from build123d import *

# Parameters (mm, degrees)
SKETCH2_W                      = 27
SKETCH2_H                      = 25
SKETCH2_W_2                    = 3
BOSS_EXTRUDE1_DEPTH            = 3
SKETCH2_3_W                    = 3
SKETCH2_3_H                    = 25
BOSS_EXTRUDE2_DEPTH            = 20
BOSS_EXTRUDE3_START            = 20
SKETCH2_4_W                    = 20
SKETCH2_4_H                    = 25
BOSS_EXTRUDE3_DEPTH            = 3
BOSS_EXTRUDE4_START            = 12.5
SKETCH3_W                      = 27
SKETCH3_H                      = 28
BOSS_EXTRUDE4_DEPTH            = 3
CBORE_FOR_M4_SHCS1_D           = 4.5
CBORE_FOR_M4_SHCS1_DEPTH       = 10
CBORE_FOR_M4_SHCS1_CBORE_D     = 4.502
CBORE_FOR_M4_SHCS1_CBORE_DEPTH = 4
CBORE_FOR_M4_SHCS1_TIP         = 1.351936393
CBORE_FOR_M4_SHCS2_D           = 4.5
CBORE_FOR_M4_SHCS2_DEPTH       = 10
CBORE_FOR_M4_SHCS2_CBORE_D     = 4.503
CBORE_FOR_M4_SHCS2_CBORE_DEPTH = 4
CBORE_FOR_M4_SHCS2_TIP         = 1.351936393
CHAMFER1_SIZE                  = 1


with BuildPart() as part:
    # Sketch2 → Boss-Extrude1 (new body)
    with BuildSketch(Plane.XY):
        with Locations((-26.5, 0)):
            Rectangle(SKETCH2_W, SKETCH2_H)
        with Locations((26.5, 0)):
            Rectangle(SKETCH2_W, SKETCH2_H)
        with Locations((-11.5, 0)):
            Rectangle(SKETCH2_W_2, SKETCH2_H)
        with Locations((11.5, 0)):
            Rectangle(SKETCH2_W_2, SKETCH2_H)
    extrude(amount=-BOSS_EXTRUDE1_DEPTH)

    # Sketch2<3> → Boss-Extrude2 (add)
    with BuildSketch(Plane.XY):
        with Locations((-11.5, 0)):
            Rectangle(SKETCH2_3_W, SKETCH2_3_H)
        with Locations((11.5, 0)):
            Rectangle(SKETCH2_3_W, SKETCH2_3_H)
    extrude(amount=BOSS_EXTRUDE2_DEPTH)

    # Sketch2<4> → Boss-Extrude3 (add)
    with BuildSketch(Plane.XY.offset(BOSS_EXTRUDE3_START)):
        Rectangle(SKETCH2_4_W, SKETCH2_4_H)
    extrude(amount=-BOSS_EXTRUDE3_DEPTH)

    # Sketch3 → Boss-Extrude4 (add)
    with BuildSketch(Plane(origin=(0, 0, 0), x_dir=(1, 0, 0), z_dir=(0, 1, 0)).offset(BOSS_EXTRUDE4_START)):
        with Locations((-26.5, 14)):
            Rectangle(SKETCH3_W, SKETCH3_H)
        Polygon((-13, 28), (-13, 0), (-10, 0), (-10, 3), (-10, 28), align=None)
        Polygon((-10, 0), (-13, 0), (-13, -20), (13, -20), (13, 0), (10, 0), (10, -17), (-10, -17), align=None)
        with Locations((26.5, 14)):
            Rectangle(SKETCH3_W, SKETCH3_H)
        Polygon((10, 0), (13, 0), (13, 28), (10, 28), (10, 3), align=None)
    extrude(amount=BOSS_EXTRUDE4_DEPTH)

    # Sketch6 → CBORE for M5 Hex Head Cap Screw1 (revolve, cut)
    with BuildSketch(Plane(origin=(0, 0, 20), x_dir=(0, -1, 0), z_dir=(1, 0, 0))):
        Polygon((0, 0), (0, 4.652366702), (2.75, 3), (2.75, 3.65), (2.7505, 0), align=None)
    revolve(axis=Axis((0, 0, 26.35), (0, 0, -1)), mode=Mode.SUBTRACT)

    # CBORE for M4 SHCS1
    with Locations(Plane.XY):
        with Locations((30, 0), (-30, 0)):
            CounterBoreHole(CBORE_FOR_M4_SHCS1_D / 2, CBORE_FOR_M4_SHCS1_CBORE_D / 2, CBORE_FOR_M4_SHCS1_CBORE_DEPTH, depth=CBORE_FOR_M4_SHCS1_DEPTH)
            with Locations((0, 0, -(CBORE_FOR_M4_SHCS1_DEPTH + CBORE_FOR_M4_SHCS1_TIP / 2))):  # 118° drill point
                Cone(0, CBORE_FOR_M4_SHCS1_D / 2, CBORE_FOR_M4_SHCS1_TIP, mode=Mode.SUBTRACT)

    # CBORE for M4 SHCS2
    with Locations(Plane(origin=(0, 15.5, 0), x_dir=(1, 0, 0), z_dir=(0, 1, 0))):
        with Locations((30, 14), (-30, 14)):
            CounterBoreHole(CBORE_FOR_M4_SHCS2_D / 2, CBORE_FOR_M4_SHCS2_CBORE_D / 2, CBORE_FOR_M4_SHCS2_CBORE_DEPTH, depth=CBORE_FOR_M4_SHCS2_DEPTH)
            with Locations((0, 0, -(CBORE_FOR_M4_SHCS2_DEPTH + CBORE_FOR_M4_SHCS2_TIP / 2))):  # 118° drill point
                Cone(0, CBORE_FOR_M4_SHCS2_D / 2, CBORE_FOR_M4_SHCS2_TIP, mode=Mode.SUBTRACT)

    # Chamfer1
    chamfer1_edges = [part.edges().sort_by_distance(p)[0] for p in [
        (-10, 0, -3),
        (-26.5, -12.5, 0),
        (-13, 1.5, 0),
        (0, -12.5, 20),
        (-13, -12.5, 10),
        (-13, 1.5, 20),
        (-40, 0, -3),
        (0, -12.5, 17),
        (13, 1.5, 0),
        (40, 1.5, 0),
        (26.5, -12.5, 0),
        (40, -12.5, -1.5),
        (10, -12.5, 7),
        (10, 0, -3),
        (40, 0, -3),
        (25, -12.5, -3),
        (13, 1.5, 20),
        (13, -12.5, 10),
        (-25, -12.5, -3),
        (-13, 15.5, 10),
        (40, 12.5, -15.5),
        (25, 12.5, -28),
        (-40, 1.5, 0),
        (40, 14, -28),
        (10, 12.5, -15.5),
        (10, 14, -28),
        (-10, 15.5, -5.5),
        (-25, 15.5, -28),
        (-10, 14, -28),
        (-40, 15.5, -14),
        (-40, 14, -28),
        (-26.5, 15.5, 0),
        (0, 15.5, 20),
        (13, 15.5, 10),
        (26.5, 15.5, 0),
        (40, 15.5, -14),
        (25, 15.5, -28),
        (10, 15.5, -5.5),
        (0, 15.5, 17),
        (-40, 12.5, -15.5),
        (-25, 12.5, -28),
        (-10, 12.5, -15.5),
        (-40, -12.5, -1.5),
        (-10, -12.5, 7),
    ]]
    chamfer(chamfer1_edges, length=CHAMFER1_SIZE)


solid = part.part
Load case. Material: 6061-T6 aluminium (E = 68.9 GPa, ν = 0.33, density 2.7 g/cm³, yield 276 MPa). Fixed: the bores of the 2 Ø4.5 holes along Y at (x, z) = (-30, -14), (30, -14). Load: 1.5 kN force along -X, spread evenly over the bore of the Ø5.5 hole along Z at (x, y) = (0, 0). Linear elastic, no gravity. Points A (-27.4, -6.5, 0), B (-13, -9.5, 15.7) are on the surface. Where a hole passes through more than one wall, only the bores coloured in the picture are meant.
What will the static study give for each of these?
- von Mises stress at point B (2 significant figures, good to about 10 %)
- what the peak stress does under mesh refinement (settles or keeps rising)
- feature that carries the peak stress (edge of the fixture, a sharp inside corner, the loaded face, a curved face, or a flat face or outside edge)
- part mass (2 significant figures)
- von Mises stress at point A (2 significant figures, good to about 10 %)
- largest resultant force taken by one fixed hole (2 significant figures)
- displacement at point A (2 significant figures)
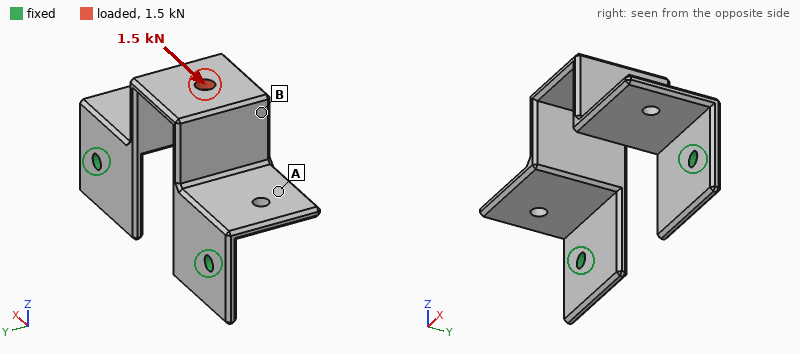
110 MPa
keeps rising
a sharp inside corner
37 g
29 MPa
1.1 kN
0.074 mm
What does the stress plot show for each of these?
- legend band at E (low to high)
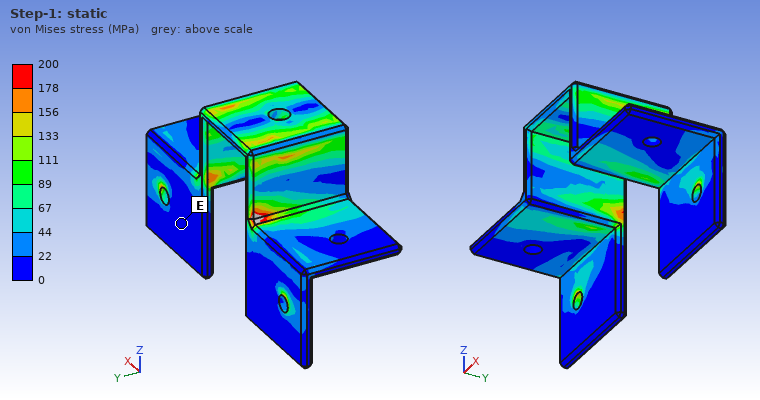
0 to 22 MPa
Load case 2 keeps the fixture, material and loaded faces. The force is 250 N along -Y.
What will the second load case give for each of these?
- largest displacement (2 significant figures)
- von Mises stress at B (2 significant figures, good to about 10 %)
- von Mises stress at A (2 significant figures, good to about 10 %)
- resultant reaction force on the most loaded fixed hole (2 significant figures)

0.57 mm
24 MPa
15 MPa
130 N
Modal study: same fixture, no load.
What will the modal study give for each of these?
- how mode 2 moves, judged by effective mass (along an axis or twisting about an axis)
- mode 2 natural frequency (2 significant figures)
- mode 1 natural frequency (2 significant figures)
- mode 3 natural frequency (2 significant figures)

along X
2800 Hz
1000 Hz
3100 Hz
